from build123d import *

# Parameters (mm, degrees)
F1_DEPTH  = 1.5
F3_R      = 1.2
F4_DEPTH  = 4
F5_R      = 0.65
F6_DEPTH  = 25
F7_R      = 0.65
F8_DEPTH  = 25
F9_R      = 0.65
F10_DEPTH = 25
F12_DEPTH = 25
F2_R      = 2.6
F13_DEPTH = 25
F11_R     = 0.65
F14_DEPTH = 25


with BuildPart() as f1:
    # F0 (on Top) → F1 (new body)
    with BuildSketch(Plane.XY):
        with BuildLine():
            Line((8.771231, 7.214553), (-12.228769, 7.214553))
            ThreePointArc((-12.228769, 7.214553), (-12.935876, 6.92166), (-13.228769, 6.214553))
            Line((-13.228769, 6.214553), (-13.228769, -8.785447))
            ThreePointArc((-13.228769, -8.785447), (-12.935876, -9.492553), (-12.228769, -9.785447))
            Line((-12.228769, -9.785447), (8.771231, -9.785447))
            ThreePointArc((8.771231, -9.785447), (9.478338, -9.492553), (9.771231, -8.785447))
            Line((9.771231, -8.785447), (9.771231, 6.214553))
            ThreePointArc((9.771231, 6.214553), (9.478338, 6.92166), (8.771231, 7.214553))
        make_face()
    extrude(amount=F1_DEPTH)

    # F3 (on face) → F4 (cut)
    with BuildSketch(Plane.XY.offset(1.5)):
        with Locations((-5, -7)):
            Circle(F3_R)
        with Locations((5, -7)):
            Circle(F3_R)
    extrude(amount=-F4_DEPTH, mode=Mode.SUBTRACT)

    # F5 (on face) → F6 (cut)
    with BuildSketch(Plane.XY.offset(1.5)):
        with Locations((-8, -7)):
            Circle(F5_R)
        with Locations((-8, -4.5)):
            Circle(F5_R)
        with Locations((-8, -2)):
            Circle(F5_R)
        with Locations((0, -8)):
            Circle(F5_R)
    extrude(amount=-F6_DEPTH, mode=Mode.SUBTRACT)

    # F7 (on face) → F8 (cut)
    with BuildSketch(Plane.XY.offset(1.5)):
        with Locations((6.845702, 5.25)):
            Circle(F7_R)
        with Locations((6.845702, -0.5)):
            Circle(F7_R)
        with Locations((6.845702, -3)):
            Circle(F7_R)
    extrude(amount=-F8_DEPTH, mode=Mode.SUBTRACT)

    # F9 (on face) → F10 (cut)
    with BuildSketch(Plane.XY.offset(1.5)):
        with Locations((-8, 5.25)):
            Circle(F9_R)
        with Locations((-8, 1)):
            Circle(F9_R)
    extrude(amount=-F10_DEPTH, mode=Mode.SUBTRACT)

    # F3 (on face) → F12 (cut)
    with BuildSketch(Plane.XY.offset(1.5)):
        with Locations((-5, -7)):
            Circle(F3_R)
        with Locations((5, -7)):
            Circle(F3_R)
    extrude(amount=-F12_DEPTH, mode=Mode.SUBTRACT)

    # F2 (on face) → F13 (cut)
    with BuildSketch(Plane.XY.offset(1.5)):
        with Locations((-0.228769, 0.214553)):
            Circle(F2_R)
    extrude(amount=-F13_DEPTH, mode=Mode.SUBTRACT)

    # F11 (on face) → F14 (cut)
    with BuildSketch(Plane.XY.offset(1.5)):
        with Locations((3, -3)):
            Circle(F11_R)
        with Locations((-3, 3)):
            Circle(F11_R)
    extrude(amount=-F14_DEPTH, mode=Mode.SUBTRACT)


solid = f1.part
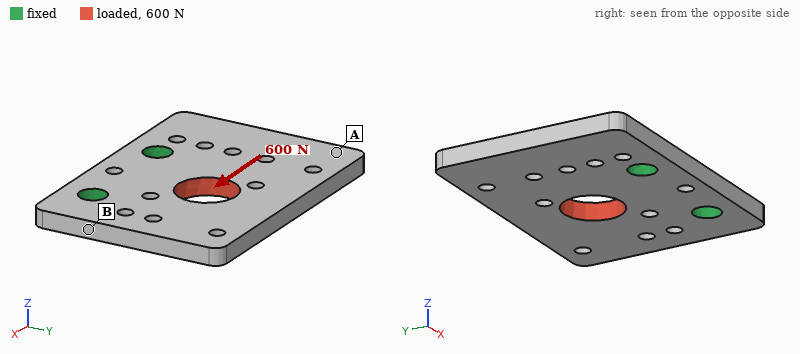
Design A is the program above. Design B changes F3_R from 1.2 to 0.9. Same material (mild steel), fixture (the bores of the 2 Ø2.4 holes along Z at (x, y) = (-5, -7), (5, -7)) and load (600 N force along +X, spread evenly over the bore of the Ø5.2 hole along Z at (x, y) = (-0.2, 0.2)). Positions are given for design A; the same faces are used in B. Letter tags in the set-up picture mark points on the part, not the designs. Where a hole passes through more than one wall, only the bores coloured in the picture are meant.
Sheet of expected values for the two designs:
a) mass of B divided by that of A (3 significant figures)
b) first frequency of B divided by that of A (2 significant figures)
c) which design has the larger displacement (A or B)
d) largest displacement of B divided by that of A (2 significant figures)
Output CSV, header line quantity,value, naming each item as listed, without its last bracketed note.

quantity,value
mass of B divided by that of A,1.01
first frequency of B divided by that of A,0.94
which design has the larger displacement,B
largest displacement of B divided by that of A,1.1
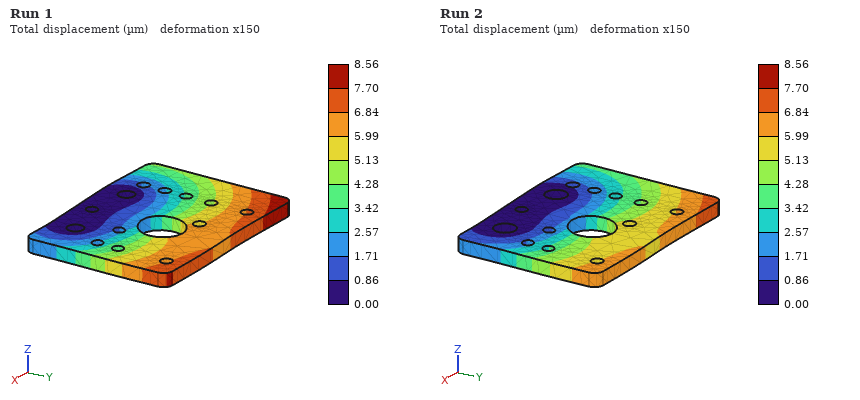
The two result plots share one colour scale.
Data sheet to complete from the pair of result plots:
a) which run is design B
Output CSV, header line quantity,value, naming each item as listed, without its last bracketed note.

quantity,value
which run is design B,Run 1
